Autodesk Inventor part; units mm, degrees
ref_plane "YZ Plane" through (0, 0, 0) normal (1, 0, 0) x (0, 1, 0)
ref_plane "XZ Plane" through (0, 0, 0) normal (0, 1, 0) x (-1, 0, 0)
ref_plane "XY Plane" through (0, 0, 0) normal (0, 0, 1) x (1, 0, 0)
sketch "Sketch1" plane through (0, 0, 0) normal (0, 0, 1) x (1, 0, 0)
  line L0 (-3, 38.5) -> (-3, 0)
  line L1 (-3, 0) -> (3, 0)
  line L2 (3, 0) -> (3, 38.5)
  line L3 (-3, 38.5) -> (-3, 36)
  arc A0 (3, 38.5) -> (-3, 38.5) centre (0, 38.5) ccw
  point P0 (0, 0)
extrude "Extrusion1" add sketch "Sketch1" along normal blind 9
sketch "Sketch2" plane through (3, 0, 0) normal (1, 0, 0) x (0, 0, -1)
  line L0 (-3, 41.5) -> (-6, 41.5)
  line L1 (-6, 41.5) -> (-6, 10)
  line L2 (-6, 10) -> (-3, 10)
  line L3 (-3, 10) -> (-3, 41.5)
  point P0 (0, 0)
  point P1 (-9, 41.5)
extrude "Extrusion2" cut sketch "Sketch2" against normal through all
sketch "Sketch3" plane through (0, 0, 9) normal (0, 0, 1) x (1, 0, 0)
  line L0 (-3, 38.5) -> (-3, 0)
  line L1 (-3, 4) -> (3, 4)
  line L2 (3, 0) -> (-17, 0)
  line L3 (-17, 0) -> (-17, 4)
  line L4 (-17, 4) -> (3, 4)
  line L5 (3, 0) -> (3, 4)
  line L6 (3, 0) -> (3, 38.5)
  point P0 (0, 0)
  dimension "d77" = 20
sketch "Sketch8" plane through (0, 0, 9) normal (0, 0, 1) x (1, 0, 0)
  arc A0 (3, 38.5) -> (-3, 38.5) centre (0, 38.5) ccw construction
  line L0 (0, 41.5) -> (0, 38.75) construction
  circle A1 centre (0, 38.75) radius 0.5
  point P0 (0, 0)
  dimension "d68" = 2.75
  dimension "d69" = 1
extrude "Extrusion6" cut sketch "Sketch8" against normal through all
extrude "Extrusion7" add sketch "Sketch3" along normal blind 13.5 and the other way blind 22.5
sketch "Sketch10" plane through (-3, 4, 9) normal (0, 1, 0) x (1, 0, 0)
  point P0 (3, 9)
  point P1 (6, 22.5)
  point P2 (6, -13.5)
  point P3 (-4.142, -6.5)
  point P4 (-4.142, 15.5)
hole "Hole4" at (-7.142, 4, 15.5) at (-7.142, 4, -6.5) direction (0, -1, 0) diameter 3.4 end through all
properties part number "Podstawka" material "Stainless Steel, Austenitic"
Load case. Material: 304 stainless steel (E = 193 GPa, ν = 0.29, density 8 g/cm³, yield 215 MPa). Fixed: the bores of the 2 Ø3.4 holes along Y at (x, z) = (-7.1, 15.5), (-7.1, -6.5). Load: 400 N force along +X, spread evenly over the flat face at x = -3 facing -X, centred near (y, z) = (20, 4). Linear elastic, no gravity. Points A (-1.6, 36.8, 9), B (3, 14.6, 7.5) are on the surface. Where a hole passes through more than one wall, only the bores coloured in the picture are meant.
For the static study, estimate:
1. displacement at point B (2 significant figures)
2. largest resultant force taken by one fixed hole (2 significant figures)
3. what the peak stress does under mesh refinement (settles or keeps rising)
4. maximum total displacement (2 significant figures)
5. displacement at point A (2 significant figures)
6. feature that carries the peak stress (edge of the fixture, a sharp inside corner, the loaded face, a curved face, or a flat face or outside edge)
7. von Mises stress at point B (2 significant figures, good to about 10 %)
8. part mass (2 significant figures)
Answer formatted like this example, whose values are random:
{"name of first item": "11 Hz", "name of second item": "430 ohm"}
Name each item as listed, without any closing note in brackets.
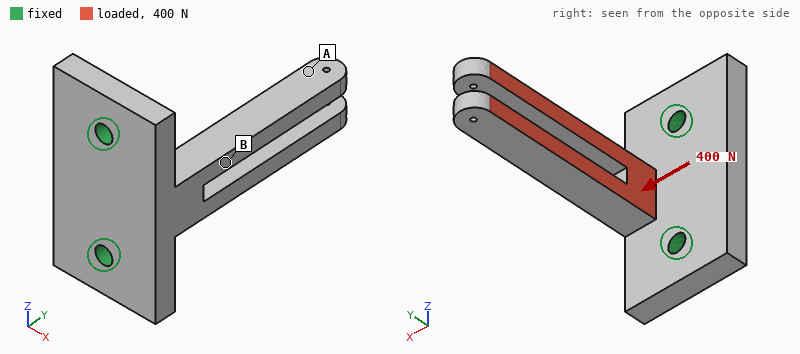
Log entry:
{"displacement at point B": "0.045 mm", "largest resultant force taken by one fixed hole": "200 N", "what the peak stress does under mesh refinement": "keeps rising", "maximum total displacement": "0.18 mm", "displacement at point A": "0.15 mm", "feature that carries the peak stress": "edge of the fixture", "von Mises stress at point B": "84 MPa", "part mass": "34 g"}
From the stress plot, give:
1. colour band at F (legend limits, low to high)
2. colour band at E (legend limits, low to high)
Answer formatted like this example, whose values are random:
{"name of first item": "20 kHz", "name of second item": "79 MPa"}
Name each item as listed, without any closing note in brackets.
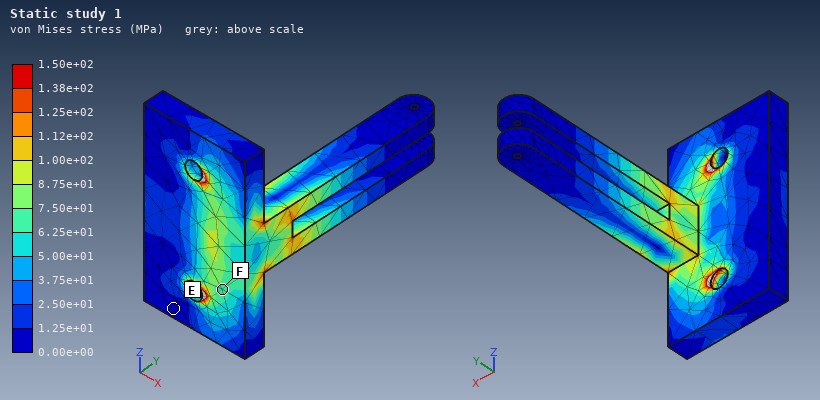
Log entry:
{"colour band at F": "6.25e+01 to 7.50e+01 MPa", "colour band at E": "0.00e+00 to 1.25e+01 MPa"}
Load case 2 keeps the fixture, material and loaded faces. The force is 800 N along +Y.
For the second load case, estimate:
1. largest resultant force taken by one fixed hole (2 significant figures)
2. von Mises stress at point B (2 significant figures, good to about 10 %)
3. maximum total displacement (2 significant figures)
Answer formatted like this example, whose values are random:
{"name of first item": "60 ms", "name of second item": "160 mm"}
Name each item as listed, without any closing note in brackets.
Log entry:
{"largest resultant force taken by one fixed hole": "400 N", "von Mises stress at point B": "28 MPa", "maximum total displacement": "35 µm"}
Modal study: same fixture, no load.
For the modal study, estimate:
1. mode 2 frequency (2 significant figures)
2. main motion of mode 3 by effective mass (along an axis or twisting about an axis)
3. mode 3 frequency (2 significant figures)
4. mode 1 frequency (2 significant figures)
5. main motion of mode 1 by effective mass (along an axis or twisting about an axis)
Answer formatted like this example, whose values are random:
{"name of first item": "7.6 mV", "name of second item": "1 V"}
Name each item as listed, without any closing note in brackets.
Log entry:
{"mode 2 frequency": "2300 Hz", "main motion of mode 3 by effective mass": "along X", "mode 3 frequency": "2700 Hz", "mode 1 frequency": "2100 Hz", "main motion of mode 1 by effective mass": "along Z"}
